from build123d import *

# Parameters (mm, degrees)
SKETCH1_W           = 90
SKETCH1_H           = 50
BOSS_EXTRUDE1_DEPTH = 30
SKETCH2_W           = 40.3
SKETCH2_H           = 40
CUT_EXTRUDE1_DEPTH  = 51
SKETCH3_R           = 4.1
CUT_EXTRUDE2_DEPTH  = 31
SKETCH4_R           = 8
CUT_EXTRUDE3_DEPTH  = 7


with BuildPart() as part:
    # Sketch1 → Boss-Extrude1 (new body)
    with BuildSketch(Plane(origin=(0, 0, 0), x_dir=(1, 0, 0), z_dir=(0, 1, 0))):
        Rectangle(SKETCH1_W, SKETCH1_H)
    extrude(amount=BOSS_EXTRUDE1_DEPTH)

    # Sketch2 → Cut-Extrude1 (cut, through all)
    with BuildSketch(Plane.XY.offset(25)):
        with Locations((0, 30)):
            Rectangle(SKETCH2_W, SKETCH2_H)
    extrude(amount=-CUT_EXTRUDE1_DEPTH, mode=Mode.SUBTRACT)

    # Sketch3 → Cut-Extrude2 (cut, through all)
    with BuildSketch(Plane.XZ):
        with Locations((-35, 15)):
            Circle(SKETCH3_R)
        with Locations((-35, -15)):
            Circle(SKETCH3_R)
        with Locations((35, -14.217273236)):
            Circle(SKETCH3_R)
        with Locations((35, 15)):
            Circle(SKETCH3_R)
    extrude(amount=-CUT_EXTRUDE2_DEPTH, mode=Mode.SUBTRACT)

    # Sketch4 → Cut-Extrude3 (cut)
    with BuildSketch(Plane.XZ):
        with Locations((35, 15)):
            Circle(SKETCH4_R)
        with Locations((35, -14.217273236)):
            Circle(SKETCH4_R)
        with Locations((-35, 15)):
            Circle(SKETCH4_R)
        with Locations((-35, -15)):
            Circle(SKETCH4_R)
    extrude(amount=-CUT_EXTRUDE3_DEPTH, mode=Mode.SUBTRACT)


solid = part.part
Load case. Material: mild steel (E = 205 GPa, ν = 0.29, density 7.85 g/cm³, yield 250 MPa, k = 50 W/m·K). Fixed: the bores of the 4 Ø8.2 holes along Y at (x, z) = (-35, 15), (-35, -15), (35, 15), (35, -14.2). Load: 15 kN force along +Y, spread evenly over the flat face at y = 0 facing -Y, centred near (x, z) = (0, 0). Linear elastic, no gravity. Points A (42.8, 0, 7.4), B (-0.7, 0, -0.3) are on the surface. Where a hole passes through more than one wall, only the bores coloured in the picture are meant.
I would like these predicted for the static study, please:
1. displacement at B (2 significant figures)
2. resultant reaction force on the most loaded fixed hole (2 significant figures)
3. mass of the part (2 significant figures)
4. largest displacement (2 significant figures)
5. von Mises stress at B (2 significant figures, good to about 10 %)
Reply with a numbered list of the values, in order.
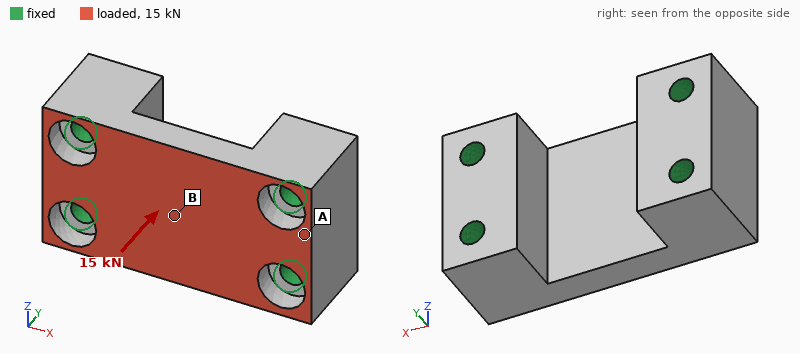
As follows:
1. 6.6 µm
2. 4.2 kN
3. 660 g
4. 7.4 µm
5. 28 MPa
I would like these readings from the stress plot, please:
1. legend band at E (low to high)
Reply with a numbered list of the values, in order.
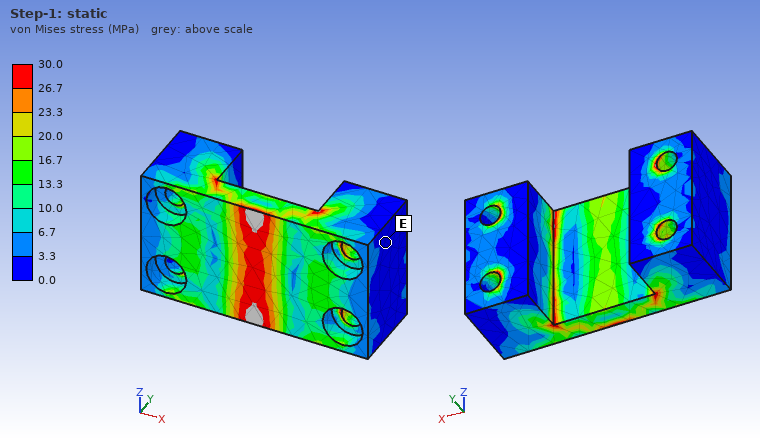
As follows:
1. 0.0 to 3.3 MPa
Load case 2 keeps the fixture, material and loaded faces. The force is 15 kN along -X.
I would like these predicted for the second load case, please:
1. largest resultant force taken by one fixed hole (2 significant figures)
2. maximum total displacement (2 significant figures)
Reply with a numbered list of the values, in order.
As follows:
1. 4.0 kN
2. 3.0 µm
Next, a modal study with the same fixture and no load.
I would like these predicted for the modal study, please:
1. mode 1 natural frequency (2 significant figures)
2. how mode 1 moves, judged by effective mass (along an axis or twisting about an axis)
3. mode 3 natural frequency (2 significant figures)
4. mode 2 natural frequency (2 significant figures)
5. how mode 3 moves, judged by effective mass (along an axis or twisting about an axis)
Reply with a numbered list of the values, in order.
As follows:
1. 15 kHz
2. along Y
3. 21 kHz
4. 18 kHz
5. along Z
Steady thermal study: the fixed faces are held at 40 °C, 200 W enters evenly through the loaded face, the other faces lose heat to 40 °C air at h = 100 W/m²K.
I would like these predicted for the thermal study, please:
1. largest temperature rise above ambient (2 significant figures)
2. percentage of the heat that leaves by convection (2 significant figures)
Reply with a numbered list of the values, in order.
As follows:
1. 57 K
2. 11 %
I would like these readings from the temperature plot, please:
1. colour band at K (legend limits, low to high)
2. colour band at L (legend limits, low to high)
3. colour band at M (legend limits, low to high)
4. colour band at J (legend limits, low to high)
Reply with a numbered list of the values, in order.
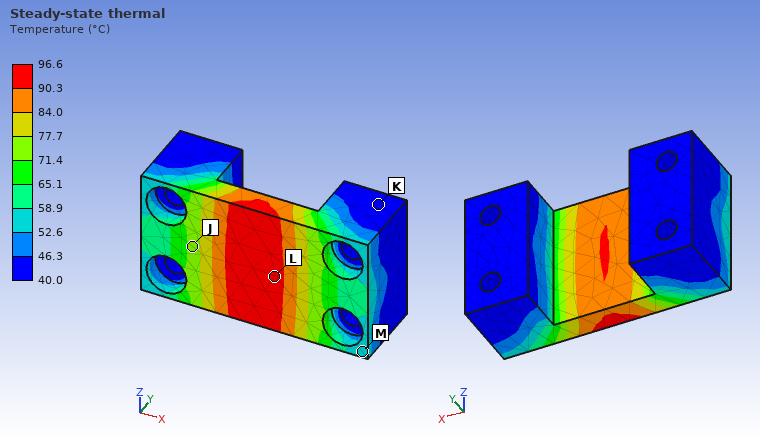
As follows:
1. 40.0 to 46.3 °C
2. 90.3 to 96.6 °C
3. 52.6 to 58.9 °C
4. 71.4 to 77.7 °C
